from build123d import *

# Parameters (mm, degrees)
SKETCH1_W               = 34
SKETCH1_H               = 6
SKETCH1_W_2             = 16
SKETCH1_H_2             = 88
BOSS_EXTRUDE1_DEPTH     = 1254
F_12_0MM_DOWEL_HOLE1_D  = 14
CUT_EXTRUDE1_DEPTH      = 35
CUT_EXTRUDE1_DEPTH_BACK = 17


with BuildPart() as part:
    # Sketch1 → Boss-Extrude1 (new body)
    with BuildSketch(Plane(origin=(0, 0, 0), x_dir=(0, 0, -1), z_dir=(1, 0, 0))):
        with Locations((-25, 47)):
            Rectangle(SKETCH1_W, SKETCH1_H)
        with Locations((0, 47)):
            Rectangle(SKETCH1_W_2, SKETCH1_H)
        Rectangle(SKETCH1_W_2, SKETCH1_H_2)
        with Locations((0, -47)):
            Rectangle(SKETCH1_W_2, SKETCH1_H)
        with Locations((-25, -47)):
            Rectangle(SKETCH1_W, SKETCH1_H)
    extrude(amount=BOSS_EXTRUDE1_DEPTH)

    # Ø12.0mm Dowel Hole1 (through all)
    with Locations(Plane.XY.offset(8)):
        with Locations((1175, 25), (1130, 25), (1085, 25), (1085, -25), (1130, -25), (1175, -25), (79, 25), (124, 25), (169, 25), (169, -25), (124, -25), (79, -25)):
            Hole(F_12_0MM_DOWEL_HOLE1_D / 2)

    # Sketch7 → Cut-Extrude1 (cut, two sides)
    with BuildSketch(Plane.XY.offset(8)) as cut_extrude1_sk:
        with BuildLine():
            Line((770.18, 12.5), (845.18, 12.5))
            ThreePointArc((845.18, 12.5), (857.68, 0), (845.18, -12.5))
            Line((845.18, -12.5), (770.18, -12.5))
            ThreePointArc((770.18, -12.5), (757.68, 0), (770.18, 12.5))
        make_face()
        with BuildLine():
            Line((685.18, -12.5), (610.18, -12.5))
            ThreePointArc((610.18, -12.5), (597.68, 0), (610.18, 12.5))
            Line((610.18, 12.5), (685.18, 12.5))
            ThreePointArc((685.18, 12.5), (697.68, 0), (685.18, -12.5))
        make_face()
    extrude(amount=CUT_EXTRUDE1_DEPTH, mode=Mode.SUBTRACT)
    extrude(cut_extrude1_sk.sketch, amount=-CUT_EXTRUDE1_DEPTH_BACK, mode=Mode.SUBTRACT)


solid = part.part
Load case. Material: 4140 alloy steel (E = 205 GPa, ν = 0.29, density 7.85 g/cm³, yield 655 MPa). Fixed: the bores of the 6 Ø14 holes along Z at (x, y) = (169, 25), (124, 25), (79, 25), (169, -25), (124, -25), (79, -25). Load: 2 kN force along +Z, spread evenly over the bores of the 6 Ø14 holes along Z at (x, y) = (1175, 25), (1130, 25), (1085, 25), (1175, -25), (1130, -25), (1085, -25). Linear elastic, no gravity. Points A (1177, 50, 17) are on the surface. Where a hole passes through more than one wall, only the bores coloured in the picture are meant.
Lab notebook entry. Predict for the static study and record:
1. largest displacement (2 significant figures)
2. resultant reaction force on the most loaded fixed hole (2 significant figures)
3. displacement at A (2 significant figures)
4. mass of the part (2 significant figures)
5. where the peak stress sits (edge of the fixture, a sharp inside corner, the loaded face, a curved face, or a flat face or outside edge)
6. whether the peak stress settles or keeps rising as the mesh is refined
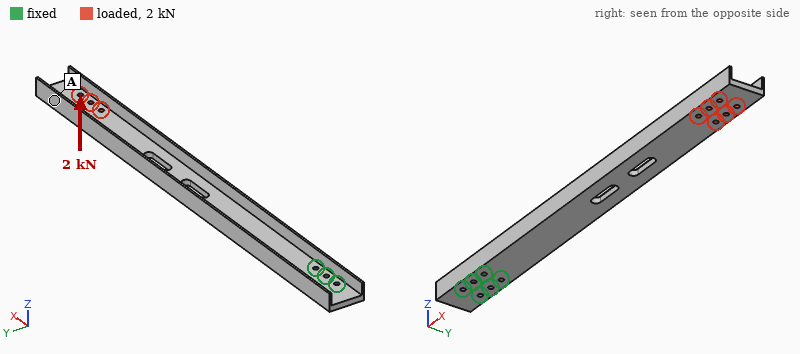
14 mm
16 kN
12 mm
19 kg
edge of the fixture
keeps rising
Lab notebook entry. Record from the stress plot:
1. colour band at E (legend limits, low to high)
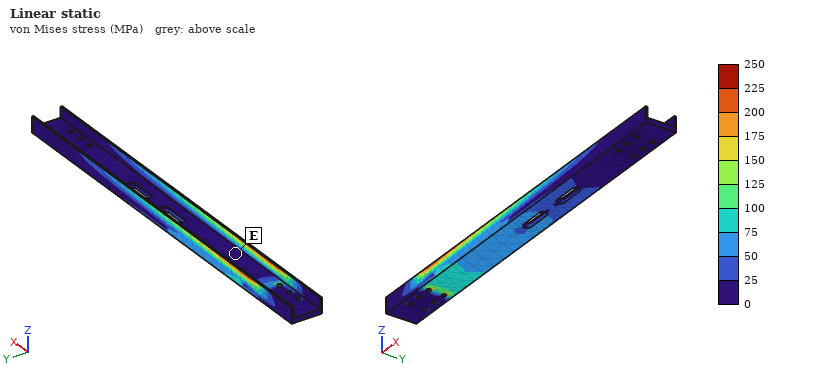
0 to 25 MPa
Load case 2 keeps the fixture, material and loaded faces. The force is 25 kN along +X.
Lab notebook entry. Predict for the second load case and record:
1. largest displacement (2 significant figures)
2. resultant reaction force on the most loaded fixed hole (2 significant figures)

1.4 mm
11 kN
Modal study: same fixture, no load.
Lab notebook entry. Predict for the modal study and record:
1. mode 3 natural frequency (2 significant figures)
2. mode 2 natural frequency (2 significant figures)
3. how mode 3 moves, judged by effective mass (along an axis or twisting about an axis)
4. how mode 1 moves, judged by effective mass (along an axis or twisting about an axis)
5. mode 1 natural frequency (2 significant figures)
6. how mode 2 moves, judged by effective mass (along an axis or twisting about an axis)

170 Hz
77 Hz
along Z
along Z
28 Hz
along Y
